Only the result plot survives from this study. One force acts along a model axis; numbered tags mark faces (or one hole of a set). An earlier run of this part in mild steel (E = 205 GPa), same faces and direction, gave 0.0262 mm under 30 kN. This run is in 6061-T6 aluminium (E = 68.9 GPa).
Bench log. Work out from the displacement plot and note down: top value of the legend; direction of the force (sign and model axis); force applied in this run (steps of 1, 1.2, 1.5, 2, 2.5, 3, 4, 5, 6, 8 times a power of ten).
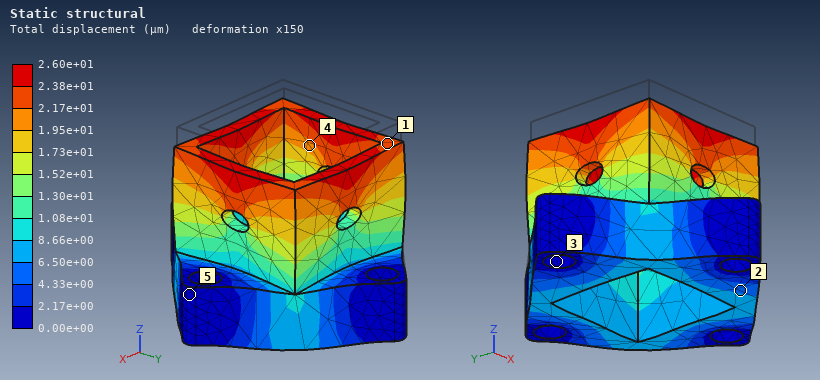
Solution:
2.60e+01 µm
-Z
10 kN
